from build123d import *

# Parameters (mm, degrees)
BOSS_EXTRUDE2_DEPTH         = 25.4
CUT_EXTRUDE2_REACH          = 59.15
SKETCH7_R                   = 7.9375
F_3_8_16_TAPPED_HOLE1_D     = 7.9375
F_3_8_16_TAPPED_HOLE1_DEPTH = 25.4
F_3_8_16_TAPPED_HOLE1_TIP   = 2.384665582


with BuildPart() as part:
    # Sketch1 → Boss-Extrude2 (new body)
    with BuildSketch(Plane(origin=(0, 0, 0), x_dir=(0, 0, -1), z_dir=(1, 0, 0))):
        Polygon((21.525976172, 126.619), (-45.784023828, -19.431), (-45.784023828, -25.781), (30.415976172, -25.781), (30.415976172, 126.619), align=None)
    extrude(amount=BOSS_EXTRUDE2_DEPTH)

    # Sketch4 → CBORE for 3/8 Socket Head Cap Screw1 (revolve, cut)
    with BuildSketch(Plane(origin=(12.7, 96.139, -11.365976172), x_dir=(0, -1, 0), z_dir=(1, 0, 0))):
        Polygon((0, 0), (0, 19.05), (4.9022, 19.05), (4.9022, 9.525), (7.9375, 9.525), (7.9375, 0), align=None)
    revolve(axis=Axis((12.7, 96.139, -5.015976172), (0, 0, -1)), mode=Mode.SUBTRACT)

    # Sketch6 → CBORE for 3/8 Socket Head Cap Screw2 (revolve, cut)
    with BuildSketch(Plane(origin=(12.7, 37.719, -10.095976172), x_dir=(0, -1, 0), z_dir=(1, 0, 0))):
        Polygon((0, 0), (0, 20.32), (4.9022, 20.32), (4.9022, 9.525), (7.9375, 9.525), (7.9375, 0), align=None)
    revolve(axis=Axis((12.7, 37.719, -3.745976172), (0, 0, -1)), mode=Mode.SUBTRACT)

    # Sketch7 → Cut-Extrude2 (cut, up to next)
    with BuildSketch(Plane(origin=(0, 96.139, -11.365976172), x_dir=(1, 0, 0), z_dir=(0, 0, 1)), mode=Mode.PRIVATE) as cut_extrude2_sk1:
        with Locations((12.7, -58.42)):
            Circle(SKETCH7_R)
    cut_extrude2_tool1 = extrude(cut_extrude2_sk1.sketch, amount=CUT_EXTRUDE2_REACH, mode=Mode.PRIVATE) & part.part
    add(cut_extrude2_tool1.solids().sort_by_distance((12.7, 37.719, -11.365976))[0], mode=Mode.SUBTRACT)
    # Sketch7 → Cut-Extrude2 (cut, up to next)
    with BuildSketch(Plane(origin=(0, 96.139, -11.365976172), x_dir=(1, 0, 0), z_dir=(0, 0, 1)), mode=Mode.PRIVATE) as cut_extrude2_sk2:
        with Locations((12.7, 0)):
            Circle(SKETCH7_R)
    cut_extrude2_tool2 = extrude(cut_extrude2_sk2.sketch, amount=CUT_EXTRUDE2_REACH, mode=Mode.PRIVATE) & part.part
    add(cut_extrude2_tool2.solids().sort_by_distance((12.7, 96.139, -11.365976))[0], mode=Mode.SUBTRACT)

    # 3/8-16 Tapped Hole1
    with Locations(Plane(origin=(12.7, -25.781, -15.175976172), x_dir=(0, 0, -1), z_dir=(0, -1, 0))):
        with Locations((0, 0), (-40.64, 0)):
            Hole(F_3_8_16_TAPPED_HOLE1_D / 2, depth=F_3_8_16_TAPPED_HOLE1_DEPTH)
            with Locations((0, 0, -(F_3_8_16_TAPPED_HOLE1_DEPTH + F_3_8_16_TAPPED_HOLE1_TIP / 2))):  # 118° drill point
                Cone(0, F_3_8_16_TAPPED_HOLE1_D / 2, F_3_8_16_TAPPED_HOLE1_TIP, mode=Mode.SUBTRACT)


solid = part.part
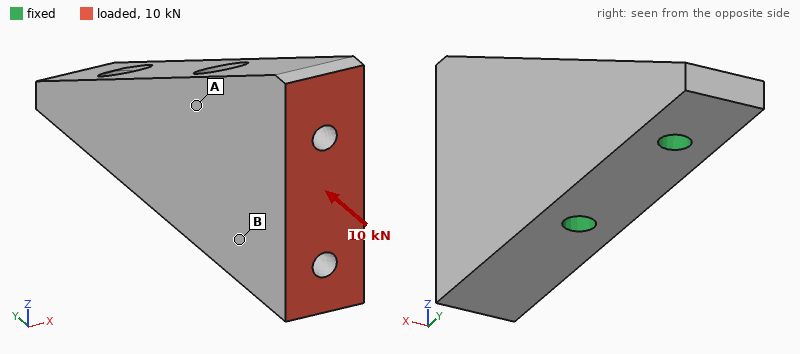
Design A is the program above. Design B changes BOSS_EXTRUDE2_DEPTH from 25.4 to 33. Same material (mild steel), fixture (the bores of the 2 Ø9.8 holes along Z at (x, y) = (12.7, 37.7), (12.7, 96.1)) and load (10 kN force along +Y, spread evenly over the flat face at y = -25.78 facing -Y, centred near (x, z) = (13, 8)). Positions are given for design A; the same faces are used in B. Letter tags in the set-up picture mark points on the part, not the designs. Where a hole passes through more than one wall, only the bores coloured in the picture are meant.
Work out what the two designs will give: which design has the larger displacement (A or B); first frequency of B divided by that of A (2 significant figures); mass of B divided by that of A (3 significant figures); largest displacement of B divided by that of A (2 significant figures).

A
1.0
1.33
0.78
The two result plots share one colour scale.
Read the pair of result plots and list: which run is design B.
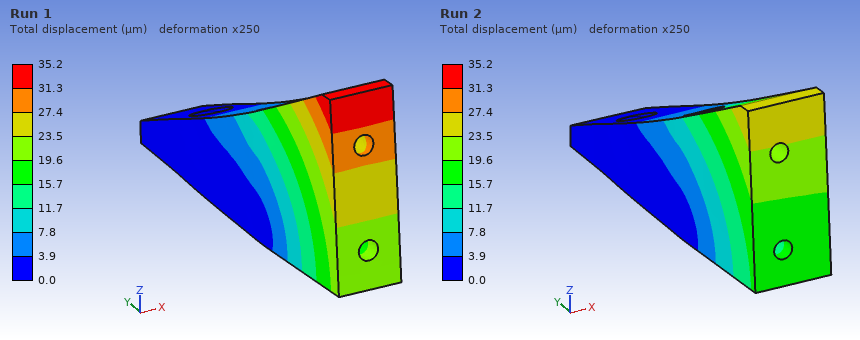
Run 2
